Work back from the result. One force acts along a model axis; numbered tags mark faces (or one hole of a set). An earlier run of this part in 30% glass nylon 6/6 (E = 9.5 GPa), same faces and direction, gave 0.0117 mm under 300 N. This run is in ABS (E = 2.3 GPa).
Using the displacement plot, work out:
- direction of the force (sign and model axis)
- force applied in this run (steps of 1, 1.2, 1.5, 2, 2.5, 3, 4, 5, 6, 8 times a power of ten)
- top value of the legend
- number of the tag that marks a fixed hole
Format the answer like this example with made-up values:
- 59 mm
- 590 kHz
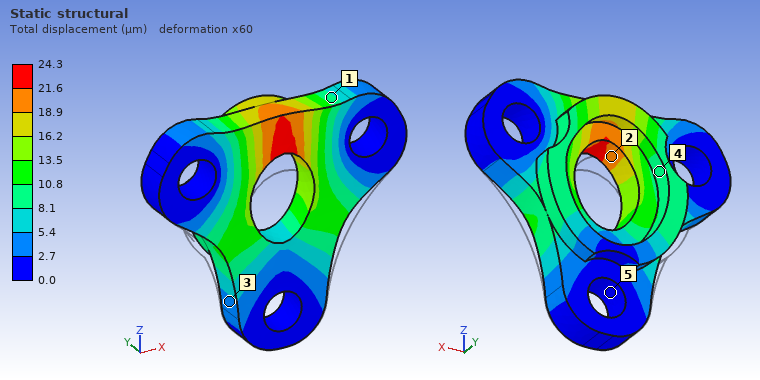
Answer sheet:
- +Z
- 150 N
- 24.3 µm
- 5
